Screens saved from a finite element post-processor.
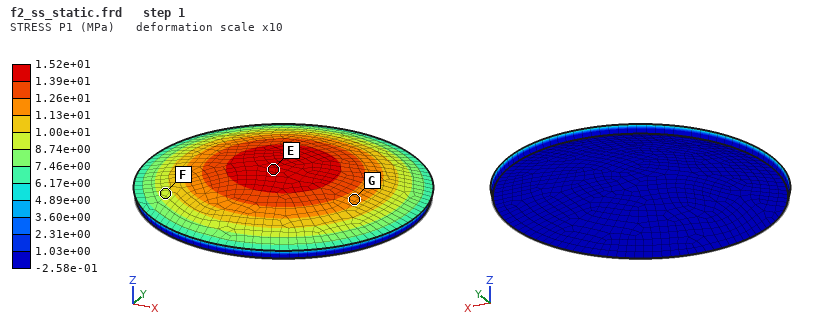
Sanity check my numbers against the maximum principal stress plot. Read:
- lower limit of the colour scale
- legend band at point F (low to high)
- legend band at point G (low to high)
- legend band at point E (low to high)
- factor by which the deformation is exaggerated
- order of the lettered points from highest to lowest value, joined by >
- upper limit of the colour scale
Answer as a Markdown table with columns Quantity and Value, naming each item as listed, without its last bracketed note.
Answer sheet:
| Quantity | Value |
|---|---|
| lower limit of the colour scale | -2.58e-01 MPa |
| legend band at point F | 8.74e+00 to 1.00e+01 MPa |
| legend band at point G | 1.13e+01 to 1.26e+01 MPa |
| legend band at point E | 1.39e+01 to 1.52e+01 MPa |
| factor by which the deformation is exaggerated | 10 |
| order of the lettered points from highest to lowest value, joined by > | E > G > F |
| upper limit of the colour scale | 1.52e+01 MPa |
